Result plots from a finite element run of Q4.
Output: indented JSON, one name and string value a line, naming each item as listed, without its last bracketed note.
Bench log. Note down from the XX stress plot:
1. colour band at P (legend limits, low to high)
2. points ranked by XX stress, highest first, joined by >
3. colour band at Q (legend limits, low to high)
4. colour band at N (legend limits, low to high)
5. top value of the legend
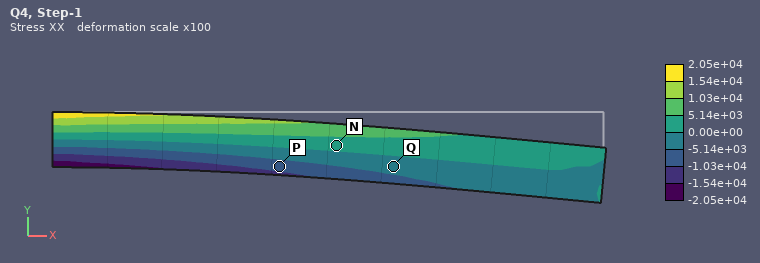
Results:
{
  "colour band at P": "-1.03e+04 to -5.14e+03",
  "points ranked by XX stress, highest first, joined by >": "N > Q > P",
  "colour band at Q": "-5.14e+03 to 0.00e+00",
  "colour band at N": "0.00e+00 to 5.14e+03",
  "top value of the legend": "2.05e+04"
}
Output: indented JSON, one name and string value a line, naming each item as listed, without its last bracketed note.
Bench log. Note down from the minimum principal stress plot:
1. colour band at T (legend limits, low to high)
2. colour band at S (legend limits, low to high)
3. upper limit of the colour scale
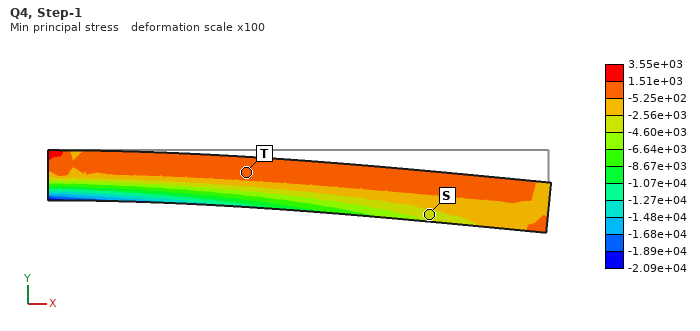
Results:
{
  "colour band at T": "-5.25e+02 to 1.51e+03",
  "colour band at S": "-4.60e+03 to -2.56e+03",
  "upper limit of the colour scale": "3.55e+03"
}
